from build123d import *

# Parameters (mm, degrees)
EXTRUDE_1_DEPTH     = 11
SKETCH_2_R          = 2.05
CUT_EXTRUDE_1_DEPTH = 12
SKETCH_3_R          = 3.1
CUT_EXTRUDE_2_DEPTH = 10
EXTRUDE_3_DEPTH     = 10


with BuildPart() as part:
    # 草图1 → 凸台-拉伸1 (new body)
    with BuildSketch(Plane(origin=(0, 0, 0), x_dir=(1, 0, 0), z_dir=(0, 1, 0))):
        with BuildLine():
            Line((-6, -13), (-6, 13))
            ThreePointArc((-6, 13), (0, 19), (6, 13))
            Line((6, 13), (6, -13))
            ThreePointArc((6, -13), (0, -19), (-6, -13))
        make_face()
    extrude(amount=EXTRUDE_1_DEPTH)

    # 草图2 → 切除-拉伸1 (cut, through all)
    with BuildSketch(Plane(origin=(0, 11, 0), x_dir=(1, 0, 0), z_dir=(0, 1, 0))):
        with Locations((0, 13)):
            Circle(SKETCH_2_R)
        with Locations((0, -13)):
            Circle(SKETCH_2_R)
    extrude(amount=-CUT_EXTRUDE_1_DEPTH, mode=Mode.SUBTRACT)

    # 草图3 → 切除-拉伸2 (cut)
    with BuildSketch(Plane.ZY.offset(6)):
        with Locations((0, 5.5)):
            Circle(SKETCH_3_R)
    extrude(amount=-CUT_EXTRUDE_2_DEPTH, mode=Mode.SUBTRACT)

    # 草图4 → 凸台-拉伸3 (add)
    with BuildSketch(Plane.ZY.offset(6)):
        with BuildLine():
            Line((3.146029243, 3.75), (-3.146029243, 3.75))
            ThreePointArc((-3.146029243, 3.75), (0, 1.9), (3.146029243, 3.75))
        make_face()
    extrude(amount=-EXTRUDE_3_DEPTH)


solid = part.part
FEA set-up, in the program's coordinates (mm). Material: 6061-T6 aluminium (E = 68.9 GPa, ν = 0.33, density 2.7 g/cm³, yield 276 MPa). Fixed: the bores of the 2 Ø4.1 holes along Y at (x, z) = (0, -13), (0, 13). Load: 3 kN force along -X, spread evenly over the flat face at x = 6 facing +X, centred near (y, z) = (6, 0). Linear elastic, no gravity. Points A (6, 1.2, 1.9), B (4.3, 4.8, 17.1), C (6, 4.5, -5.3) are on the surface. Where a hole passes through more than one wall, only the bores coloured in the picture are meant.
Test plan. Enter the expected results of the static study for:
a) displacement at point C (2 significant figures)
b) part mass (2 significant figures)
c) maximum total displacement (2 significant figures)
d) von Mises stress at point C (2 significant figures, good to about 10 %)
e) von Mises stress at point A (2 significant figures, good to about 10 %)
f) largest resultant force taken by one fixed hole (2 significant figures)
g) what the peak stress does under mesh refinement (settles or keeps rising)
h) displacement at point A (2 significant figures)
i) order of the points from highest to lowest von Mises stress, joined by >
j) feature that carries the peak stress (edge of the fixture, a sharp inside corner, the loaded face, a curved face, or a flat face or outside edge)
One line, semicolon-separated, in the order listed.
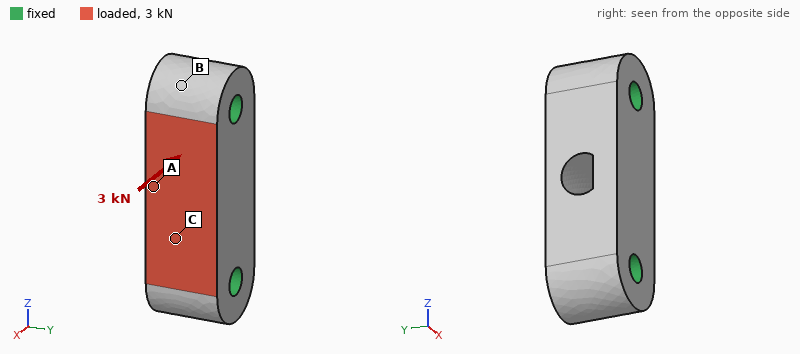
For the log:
4.8 µm; 11 g; 6.7 µm; 13 MPa; 23 MPa; 1.5 kN; keeps rising; 5.7 µm; A > C > B; edge of the fixture
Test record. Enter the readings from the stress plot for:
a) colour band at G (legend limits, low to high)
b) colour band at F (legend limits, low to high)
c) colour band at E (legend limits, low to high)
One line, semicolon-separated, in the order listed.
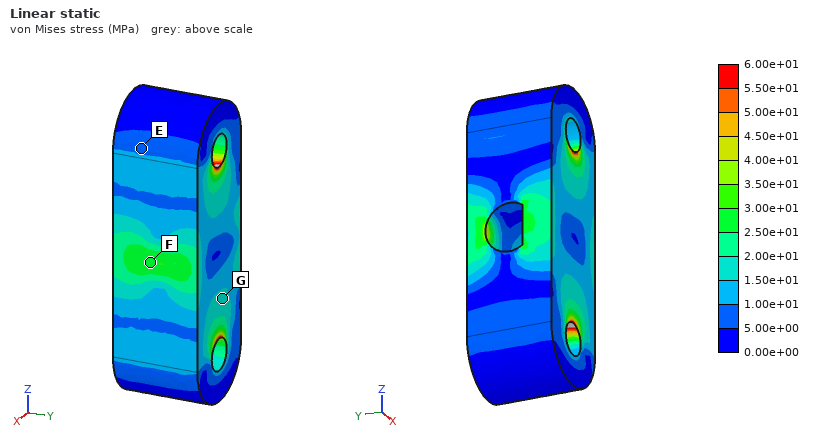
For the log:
1.50e+01 to 2.00e+01 MPa; 2.50e+01 to 3.00e+01 MPa; 5.00e+00 to 1.00e+01 MPa
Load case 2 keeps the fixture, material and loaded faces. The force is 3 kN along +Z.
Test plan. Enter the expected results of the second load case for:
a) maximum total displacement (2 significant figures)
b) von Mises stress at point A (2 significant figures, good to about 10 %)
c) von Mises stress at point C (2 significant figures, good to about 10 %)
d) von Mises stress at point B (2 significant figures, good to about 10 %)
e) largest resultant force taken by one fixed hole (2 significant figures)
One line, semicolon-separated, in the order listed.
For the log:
3.1 µm; 18 MPa; 20 MPa; 5.6 MPa; 1.6 kN
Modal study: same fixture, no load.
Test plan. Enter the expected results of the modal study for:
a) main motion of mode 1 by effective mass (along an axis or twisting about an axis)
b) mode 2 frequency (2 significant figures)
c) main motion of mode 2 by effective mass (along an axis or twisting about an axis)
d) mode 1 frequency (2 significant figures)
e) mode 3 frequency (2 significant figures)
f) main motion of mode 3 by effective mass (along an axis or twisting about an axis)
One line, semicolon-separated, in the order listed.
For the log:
along X; 52 kHz; along Y; 46 kHz; 58 kHz; twisting about Z
